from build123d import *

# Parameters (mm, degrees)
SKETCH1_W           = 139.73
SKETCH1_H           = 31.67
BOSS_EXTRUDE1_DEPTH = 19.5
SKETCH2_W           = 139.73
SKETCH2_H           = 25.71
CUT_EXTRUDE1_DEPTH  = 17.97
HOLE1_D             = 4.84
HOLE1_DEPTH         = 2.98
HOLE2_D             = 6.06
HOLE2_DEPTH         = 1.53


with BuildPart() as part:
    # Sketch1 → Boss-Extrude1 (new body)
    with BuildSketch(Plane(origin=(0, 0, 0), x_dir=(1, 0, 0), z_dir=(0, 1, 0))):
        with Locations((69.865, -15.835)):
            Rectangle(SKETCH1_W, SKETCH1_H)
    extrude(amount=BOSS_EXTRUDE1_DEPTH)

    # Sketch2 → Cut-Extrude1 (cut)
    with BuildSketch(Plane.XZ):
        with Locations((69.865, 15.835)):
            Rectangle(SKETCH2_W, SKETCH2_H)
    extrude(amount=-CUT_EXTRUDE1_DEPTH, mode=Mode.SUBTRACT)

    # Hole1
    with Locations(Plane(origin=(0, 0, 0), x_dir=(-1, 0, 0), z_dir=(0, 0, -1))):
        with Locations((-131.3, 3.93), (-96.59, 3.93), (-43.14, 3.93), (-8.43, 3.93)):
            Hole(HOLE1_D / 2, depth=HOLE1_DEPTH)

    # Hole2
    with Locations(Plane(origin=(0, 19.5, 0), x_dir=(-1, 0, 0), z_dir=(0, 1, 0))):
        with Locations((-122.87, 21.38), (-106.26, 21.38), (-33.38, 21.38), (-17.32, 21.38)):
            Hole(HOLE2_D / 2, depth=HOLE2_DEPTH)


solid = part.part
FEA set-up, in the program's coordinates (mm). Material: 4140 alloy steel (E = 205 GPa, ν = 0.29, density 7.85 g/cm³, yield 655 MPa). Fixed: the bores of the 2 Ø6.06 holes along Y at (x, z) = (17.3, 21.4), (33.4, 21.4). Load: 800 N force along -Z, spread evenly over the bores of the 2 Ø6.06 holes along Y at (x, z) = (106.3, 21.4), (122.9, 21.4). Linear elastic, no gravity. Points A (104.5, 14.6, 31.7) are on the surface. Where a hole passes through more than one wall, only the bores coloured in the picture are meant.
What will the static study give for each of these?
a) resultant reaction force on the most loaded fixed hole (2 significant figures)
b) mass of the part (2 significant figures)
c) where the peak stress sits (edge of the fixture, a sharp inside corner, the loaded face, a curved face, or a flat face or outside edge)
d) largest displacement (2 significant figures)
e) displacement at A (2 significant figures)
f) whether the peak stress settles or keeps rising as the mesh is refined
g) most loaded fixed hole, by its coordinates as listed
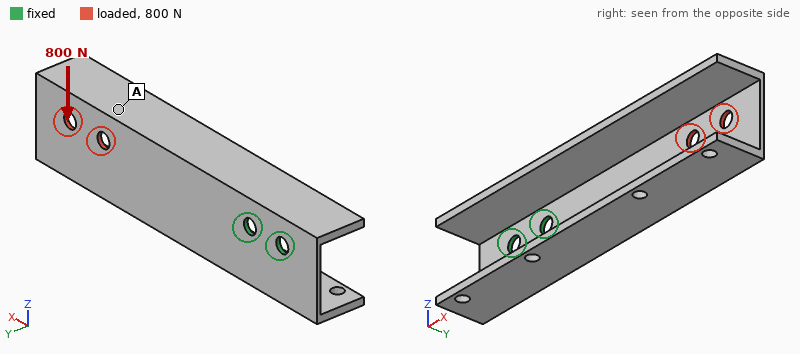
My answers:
3.5 kN
170 g
edge of the fixture
0.28 mm
0.17 mm
keeps rising
(33.4, 21.4)
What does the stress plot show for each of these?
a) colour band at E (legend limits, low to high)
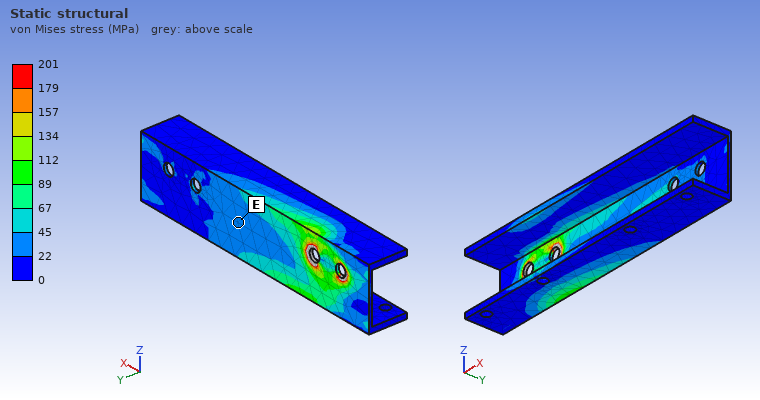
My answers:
22 to 45 MPa
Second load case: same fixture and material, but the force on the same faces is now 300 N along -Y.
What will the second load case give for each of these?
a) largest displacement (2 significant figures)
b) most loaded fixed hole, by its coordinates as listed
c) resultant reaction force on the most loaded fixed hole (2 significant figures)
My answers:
0.66 mm
(33.4, 21.4)
1.5 kN
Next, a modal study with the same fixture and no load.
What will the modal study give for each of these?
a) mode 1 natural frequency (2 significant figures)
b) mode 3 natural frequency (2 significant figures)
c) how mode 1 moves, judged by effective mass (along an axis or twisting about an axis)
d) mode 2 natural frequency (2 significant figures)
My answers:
400 Hz
1200 Hz
along Y
630 Hz
